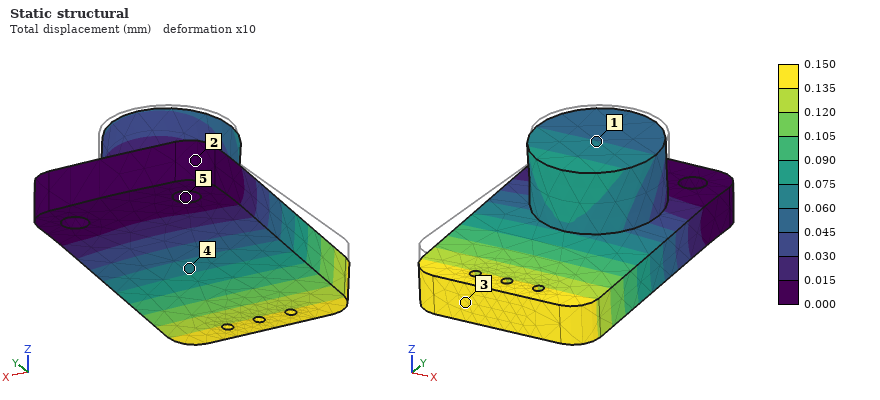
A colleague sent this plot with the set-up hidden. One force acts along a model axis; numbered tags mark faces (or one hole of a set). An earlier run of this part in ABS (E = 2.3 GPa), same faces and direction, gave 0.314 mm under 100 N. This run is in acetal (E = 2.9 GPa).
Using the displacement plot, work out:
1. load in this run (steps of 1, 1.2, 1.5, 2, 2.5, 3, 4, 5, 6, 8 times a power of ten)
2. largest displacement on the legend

60 N
0.150 mm
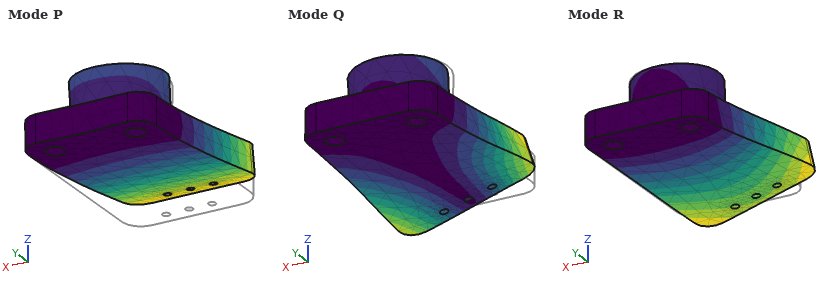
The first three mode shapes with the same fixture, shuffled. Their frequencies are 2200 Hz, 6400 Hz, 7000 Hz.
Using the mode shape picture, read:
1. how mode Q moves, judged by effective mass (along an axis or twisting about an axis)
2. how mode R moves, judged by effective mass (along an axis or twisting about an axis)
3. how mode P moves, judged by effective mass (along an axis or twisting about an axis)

along X
along X
along Z
